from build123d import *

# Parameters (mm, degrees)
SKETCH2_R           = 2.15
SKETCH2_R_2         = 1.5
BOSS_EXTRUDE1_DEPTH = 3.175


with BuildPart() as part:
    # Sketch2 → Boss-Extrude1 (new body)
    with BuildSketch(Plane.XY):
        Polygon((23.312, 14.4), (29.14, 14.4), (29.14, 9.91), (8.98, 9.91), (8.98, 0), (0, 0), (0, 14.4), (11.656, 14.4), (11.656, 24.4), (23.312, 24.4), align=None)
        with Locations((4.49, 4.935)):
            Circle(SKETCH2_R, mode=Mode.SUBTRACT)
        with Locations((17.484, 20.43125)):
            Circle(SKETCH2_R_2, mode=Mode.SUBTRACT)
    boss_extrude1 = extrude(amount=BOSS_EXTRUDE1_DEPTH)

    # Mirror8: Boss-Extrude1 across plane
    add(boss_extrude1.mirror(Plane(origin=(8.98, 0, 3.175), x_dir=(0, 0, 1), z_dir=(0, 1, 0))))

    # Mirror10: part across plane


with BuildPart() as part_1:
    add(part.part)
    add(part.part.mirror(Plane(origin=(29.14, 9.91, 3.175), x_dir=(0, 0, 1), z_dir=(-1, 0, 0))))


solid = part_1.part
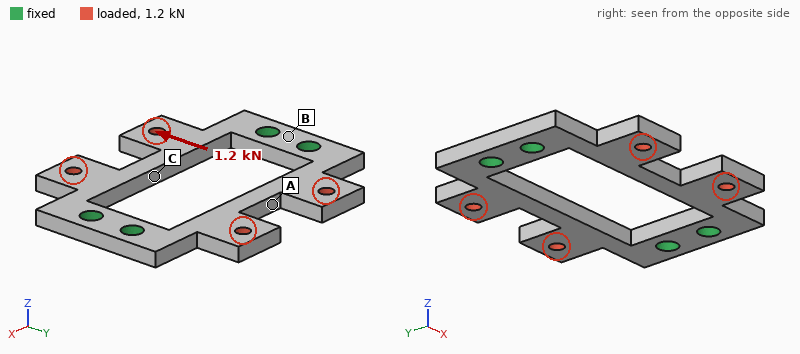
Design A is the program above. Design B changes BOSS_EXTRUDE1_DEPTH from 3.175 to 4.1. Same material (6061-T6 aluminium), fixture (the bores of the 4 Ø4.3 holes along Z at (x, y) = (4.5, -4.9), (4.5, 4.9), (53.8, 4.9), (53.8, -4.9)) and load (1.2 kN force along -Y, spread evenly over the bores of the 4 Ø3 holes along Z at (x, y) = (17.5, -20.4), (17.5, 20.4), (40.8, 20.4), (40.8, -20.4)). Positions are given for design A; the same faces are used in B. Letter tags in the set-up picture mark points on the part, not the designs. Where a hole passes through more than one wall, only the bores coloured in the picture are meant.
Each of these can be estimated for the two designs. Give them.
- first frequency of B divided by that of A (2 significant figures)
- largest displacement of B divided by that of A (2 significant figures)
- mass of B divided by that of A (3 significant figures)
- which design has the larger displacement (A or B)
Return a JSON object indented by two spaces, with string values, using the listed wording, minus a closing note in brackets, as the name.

{
  "first frequency of B divided by that of A": "1.3",
  "largest displacement of B divided by that of A": "0.76",
  "mass of B divided by that of A": "1.29",
  "which design has the larger displacement": "A"
}
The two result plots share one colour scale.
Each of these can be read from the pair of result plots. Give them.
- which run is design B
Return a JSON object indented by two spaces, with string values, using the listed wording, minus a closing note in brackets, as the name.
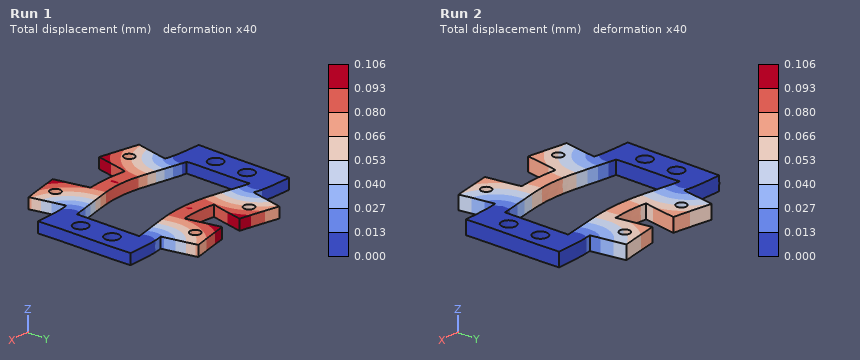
{
  "which run is design B": "Run 2"
}
